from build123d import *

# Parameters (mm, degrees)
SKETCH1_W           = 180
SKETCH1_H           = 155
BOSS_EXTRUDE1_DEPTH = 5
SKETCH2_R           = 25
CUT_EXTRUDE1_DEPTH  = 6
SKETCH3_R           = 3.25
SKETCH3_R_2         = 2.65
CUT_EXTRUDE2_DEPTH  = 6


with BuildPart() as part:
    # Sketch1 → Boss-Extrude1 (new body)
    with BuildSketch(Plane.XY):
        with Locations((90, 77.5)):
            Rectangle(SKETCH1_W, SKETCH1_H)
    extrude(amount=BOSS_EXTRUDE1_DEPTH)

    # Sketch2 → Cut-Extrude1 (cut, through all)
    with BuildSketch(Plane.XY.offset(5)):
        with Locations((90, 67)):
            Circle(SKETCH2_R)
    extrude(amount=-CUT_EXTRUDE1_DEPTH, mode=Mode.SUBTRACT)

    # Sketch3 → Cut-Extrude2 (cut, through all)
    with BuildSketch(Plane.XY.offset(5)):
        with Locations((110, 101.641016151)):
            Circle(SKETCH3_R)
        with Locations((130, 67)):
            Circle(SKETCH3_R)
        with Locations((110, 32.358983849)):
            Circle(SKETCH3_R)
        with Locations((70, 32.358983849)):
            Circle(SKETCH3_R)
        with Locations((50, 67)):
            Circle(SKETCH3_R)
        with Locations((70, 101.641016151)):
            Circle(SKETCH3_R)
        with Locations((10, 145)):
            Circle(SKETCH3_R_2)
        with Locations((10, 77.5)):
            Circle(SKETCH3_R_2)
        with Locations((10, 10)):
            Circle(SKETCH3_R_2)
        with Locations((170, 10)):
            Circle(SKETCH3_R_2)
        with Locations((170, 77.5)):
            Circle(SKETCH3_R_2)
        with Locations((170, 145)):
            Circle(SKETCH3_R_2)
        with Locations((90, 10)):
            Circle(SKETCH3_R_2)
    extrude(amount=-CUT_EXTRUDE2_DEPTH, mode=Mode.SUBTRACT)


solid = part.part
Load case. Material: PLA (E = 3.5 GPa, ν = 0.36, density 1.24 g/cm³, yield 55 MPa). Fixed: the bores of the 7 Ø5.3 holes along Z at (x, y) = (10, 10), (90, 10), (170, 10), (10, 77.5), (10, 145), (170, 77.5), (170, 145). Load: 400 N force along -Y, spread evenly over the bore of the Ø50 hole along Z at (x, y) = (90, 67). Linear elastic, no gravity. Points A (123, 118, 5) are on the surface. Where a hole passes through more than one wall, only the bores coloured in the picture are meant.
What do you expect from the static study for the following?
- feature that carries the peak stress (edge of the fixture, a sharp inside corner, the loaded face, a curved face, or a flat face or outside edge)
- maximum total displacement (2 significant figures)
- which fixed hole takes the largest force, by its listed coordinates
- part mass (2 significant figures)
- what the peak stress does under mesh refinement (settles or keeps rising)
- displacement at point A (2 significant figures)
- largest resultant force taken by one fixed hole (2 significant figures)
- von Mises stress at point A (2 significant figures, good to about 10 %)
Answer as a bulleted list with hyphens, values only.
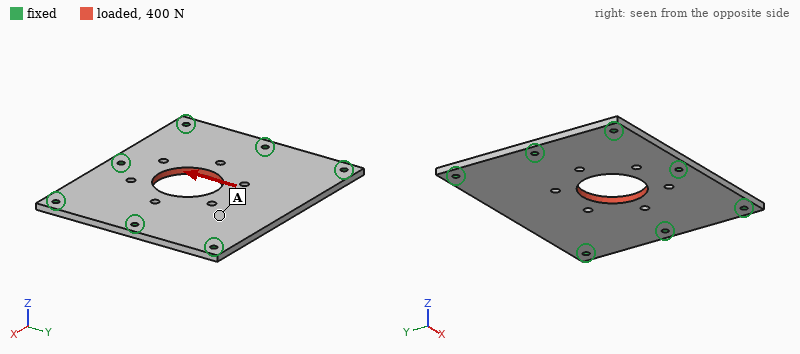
- edge of the fixture
- 17 µm
- (90, 10)
- 160 g
- keeps rising
- 9.6 µm
- 130 N
- 0.39 MPa
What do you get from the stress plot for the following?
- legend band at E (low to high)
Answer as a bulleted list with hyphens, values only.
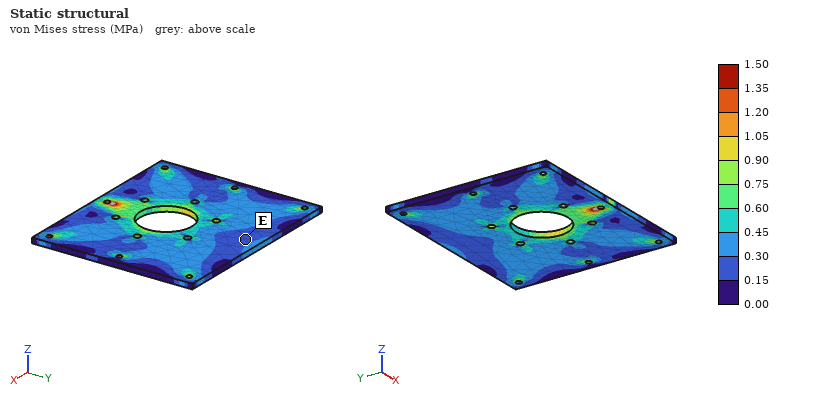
- 0.15 to 0.30 MPa
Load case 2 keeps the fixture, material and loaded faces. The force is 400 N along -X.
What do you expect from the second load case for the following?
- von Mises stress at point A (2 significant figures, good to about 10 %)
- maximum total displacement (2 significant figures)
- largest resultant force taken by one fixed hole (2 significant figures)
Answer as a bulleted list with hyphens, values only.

- 0.19 MPa
- 11 µm
- 85 N
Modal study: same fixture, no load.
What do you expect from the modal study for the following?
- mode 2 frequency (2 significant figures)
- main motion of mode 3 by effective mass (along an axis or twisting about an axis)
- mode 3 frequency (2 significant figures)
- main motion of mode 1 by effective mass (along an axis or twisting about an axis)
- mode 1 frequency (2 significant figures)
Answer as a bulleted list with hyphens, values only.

- 660 Hz
- twisting about Y
- 820 Hz
- along Z
- 340 Hz
